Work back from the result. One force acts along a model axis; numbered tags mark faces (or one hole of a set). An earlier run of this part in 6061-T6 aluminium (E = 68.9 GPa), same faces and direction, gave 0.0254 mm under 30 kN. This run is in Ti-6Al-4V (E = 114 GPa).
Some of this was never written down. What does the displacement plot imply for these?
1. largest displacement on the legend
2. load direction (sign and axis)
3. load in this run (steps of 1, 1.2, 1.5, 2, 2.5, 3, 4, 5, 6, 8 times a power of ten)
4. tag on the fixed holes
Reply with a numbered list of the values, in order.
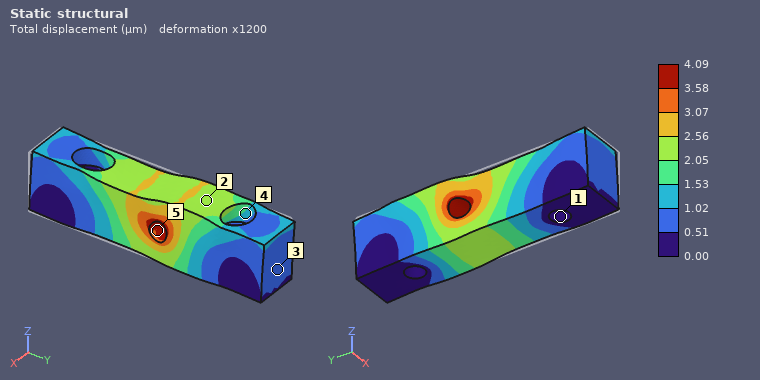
1. 4.09 µm
2. +Y
3. 8 kN
4. 1
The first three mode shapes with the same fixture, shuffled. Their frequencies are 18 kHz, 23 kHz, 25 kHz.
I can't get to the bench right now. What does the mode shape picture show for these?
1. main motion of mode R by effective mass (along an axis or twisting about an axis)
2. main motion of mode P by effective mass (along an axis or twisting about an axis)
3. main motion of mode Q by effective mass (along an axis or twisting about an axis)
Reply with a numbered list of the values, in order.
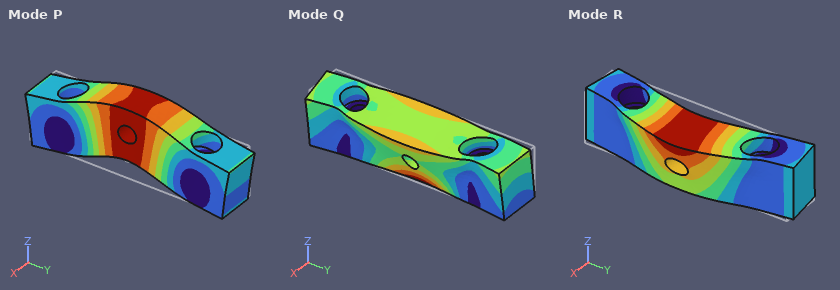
1. along X
2. along Z
3. twisting about Y
